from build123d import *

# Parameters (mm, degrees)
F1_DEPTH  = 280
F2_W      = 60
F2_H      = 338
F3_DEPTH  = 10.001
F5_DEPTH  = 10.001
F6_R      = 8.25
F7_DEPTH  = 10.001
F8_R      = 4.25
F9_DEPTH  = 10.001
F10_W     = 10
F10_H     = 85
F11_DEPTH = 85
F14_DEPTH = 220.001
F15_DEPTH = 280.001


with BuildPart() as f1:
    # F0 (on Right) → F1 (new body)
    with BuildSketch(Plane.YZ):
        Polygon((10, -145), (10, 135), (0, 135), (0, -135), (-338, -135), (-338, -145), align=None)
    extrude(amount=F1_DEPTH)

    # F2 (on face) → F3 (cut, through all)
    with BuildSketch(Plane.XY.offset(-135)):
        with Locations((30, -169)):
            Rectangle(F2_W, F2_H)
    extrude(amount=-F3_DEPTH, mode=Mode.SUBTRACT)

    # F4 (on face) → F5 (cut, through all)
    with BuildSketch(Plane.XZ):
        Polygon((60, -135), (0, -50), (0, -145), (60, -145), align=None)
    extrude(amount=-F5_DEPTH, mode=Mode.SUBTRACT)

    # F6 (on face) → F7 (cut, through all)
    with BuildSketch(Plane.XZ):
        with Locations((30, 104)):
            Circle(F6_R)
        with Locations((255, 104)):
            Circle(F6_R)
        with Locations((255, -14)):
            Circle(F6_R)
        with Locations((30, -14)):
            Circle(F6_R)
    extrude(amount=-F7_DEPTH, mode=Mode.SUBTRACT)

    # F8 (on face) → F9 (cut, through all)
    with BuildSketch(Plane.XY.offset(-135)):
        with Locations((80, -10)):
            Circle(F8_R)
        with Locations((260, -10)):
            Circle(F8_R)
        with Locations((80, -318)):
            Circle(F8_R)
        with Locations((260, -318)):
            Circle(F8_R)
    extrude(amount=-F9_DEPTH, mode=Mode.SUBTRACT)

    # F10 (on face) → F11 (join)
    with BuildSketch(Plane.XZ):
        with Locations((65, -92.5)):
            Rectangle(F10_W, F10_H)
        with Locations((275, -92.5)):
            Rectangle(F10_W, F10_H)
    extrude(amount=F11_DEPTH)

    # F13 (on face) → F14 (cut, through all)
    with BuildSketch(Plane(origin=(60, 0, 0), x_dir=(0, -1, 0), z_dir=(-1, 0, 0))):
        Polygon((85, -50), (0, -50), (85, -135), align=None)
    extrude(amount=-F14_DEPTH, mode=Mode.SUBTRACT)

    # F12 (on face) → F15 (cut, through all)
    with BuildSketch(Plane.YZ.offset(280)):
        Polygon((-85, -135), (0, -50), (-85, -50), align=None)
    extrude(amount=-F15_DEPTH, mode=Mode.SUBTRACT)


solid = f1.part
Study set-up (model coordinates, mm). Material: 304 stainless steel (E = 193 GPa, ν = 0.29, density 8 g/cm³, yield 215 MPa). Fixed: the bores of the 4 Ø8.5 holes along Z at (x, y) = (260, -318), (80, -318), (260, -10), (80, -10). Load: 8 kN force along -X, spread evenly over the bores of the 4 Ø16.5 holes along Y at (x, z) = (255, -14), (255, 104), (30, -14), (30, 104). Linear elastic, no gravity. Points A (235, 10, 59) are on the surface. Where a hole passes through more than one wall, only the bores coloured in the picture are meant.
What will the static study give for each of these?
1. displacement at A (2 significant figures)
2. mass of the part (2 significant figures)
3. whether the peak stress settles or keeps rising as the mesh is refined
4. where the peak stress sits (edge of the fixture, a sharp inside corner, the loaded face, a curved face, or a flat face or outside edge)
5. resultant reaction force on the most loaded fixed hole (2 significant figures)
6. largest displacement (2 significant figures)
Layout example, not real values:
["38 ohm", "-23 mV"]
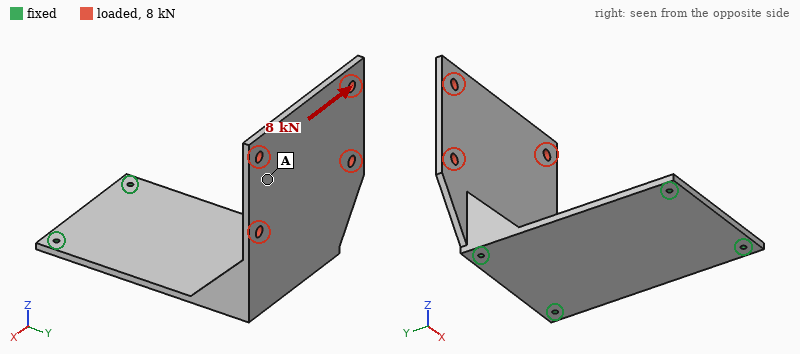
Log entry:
["0.051 mm", "12 kg", "keeps rising", "edge of the fixture", "9.1 kN", "0.14 mm"]
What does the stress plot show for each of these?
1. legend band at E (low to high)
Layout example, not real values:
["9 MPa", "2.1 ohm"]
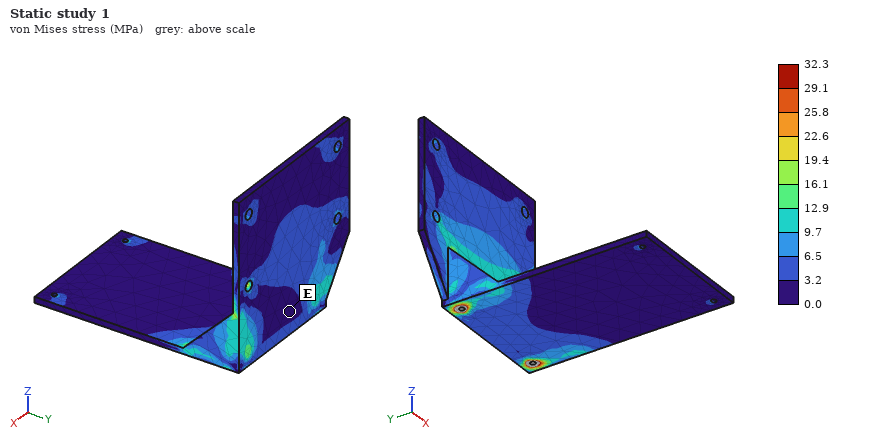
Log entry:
["0.0 to 3.2 MPa"]
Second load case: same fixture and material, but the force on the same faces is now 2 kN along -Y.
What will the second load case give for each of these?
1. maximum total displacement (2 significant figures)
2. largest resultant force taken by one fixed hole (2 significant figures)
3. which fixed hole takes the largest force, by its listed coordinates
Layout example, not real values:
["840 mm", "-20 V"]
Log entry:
["1.1 mm", "990 N", "(80, -10)"]
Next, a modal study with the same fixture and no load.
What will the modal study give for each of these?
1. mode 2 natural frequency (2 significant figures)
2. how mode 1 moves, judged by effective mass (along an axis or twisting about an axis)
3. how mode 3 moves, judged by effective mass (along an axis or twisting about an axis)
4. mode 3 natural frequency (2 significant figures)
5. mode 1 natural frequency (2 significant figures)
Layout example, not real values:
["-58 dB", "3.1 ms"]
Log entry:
["300 Hz", "along Y", "along Z", "480 Hz", "130 Hz"]
